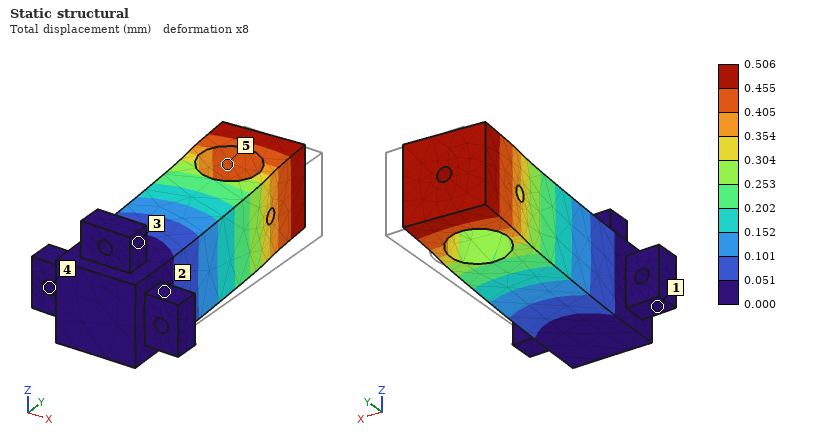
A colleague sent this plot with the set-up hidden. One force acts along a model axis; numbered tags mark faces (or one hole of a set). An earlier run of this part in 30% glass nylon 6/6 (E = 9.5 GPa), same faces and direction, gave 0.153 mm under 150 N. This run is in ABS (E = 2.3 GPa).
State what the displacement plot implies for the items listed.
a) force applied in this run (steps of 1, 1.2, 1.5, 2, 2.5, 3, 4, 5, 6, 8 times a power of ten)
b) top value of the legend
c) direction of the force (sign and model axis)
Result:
120 N
0.506 mm
-X
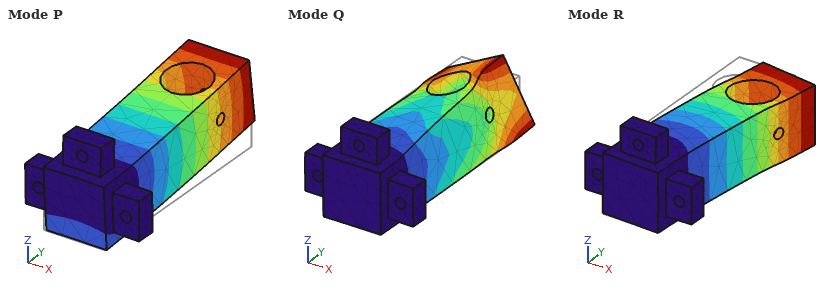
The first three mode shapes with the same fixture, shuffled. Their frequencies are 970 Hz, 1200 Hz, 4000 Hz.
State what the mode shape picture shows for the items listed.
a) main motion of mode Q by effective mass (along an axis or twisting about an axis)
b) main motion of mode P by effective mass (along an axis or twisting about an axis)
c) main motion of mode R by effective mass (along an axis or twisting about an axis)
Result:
twisting about Y
along Z
along X
